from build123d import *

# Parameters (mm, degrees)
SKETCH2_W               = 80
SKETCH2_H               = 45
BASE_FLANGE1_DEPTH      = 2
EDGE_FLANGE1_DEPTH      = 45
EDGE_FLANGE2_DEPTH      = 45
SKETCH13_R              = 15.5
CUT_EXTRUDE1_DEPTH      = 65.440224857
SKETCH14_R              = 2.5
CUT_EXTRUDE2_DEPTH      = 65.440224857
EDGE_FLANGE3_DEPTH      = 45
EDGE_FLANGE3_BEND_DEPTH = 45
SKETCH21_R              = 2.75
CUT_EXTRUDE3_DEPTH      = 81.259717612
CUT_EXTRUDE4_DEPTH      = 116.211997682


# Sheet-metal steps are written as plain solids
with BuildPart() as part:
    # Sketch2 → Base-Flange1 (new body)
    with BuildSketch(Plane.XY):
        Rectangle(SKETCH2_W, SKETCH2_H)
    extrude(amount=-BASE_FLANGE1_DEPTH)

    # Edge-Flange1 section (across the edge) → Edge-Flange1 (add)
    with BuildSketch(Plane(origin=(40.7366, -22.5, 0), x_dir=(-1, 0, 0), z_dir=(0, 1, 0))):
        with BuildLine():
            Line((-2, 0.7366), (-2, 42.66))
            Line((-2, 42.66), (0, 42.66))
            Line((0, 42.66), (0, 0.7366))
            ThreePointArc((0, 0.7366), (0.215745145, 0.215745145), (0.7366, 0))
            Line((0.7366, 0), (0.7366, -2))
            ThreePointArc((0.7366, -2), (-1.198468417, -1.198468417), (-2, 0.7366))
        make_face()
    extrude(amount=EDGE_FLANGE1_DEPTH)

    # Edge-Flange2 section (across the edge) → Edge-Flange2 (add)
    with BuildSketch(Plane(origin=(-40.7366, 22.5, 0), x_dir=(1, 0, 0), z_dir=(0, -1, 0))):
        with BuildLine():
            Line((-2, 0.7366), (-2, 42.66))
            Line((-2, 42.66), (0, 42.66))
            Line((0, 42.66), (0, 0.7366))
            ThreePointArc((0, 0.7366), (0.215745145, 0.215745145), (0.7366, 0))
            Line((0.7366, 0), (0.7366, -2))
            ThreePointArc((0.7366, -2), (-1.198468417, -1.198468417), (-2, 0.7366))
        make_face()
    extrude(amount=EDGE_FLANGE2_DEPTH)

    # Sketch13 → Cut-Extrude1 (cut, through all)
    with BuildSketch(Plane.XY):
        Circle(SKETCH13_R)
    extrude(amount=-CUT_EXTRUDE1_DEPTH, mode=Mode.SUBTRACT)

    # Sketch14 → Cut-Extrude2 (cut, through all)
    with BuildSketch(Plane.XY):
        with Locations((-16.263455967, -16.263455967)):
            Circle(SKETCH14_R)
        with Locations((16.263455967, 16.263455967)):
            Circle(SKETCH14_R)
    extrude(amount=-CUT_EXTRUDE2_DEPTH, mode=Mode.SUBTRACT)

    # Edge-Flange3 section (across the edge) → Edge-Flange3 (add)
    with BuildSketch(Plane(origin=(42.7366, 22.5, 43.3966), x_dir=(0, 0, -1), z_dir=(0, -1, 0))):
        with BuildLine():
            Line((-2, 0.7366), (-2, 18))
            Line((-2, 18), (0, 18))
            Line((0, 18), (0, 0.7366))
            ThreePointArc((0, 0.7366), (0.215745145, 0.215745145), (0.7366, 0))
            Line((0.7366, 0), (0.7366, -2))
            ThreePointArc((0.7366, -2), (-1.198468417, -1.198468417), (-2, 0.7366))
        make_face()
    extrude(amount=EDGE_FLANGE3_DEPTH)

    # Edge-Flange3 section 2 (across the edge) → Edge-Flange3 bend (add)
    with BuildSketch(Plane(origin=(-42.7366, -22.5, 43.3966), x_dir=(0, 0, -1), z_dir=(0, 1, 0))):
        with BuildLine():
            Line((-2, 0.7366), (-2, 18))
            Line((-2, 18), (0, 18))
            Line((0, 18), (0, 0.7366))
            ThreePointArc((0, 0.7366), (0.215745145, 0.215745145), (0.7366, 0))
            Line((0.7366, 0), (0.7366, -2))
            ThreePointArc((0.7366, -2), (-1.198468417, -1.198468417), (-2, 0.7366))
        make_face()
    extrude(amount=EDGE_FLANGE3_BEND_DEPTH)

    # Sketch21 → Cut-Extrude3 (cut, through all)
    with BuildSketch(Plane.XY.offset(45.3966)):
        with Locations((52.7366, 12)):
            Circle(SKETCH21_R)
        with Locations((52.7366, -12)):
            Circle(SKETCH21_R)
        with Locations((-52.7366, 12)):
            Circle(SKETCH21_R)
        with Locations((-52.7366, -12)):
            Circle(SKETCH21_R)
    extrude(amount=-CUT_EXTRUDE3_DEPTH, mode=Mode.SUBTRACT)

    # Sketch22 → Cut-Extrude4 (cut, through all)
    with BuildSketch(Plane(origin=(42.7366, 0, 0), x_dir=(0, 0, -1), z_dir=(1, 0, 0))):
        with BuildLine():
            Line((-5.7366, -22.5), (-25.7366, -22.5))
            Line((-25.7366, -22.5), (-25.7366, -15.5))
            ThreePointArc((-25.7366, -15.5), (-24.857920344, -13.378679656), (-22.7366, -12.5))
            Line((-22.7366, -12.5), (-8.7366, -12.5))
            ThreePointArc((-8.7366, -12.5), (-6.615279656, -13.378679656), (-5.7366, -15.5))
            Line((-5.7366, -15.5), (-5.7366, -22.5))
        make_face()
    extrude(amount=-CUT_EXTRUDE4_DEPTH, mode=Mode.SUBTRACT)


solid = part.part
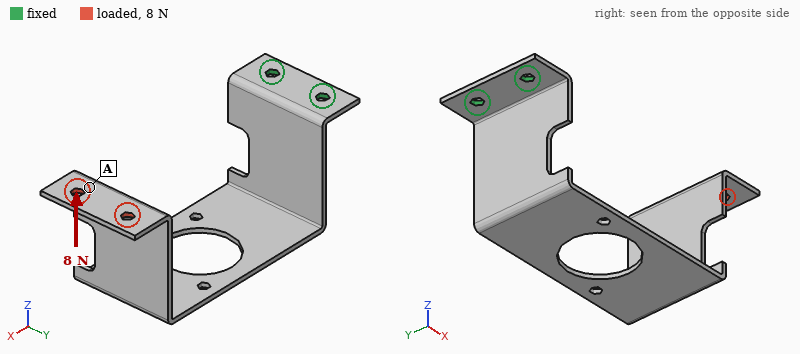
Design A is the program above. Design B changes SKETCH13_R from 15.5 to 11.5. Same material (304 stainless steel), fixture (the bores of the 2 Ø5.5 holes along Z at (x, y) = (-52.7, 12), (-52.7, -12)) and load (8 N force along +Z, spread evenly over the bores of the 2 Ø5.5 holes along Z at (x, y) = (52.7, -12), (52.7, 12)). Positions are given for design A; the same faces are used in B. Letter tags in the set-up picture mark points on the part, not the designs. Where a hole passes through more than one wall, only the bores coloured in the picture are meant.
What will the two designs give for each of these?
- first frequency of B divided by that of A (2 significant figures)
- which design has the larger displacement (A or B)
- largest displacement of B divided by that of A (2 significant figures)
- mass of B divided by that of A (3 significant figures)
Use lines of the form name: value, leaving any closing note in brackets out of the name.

first frequency of B divided by that of A: 1.0
which design has the larger displacement: A
largest displacement of B divided by that of A: 0.89
mass of B divided by that of A: 1.04
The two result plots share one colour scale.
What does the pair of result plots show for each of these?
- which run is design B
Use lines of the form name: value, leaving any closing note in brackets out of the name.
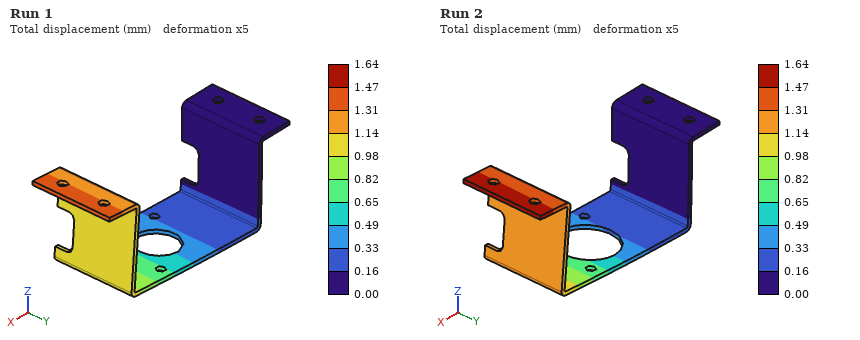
which run is design B: Run 1
